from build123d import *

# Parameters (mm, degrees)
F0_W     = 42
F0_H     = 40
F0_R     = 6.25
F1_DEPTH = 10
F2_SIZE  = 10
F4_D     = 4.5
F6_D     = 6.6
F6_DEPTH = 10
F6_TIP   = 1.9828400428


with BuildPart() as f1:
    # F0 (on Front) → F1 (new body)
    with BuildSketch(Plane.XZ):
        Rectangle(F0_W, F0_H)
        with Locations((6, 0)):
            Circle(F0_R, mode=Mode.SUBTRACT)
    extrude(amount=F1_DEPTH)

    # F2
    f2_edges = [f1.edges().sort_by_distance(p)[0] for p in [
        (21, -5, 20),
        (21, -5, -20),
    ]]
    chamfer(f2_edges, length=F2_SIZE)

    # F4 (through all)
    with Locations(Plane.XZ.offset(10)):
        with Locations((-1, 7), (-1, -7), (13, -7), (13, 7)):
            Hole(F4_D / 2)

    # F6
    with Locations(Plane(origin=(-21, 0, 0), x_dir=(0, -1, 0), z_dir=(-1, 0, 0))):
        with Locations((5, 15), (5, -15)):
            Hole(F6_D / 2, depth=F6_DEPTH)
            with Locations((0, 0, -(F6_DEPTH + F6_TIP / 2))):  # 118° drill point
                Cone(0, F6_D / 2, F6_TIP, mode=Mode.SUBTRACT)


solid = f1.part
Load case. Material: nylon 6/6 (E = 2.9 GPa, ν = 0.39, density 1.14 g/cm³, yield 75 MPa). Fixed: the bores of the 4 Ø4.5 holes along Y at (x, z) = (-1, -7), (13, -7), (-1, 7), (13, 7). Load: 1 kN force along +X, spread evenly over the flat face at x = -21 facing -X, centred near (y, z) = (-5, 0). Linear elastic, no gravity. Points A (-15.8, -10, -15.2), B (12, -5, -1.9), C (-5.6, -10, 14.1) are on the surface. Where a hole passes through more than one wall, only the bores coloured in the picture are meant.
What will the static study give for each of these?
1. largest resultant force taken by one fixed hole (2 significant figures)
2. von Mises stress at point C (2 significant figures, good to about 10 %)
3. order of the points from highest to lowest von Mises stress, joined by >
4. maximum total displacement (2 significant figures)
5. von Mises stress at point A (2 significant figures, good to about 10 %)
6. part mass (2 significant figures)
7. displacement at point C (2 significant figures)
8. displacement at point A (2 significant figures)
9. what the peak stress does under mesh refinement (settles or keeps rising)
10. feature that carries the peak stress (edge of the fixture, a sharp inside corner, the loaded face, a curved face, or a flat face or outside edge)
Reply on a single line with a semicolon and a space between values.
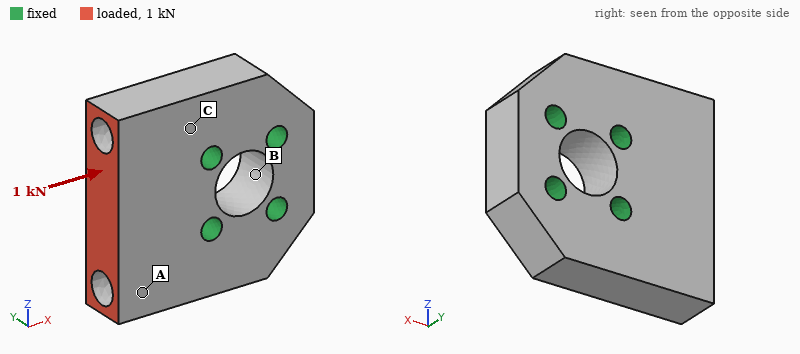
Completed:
440 N; 1.6 MPa; A > C > B; 28 µm; 3.1 MPa; 15 g; 10.0 µm; 20 µm; keeps rising; edge of the fixture
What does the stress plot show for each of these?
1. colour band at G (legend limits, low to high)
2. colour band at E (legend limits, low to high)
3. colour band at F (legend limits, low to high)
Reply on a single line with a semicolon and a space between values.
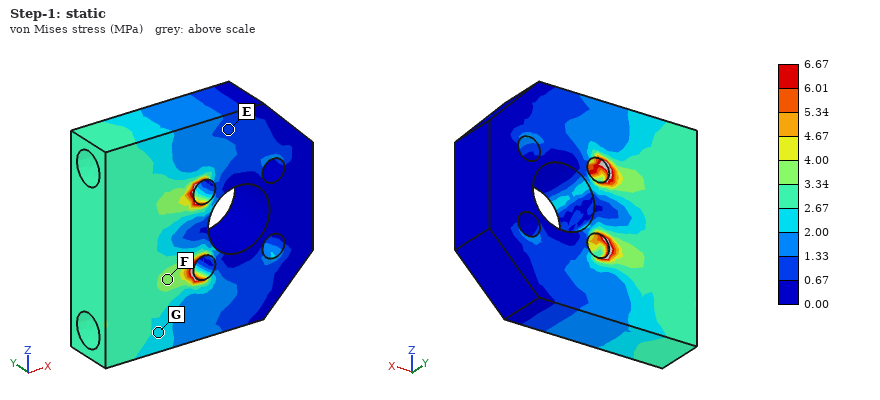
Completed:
2.00 to 2.67 MPa; 0.67 to 1.33 MPa; 3.34 to 4.00 MPa
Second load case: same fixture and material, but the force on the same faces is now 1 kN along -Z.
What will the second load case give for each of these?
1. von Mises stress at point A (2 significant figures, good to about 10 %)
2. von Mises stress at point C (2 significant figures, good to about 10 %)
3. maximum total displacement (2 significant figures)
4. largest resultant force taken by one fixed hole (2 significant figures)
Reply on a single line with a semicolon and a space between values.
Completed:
6.3 MPa; 4.3 MPa; 0.16 mm; 910 N
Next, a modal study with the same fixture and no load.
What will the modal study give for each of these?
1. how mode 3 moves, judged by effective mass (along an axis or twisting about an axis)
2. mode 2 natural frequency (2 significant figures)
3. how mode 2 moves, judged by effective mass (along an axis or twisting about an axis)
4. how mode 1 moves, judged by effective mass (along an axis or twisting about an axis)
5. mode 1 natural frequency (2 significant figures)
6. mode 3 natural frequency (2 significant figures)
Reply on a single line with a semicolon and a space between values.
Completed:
along Z; 6900 Hz; twisting about X; along Y; 5600 Hz; 8600 Hz
